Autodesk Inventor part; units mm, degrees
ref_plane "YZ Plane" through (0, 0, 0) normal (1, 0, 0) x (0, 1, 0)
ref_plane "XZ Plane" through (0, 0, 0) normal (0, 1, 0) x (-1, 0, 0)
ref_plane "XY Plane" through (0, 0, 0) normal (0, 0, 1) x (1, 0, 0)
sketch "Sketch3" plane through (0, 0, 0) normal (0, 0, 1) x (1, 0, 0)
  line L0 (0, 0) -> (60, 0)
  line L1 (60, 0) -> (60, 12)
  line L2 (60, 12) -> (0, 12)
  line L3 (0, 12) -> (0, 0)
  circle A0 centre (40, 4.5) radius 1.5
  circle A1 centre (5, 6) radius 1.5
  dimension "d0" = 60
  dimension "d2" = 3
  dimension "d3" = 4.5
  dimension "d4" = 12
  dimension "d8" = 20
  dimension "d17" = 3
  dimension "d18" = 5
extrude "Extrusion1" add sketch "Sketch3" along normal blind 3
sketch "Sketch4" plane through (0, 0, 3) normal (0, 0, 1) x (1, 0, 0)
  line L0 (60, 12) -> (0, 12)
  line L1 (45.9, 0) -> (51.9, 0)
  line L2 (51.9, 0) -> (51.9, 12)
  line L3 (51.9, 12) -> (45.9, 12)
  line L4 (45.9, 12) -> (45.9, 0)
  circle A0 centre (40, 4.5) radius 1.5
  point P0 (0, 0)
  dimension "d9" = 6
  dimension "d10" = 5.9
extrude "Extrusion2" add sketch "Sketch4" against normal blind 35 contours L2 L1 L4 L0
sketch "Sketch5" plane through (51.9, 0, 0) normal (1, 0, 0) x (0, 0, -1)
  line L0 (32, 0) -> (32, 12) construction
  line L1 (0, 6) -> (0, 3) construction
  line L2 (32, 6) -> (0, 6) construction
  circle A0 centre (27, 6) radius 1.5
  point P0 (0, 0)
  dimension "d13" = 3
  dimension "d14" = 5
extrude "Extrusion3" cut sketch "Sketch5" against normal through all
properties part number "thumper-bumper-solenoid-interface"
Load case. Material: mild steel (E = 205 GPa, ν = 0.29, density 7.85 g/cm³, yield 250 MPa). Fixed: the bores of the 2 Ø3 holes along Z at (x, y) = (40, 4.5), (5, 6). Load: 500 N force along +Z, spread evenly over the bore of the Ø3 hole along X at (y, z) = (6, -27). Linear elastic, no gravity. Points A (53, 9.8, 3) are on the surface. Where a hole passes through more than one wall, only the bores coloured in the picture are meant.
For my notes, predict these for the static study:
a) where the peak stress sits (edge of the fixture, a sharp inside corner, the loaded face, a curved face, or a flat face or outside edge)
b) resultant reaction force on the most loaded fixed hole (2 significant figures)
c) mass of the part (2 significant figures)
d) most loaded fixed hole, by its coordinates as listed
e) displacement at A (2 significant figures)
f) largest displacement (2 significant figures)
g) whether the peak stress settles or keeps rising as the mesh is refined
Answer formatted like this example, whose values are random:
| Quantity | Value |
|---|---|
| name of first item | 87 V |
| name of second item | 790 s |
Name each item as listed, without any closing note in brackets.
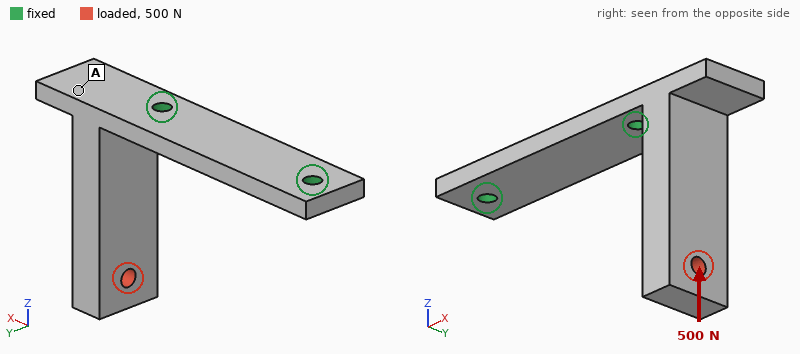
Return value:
| Quantity | Value |
|---|---|
| where the peak stress sits | edge of the fixture |
| resultant reaction force on the most loaded fixed hole | 510 N |
| mass of the part | 34 g |
| most loaded fixed hole, by its coordinates as listed | (40, 4.5) |
| displacement at A | 0.037 mm |
| largest displacement | 0.12 mm |
| whether the peak stress settles or keeps rising as the mesh is refined | keeps rising |
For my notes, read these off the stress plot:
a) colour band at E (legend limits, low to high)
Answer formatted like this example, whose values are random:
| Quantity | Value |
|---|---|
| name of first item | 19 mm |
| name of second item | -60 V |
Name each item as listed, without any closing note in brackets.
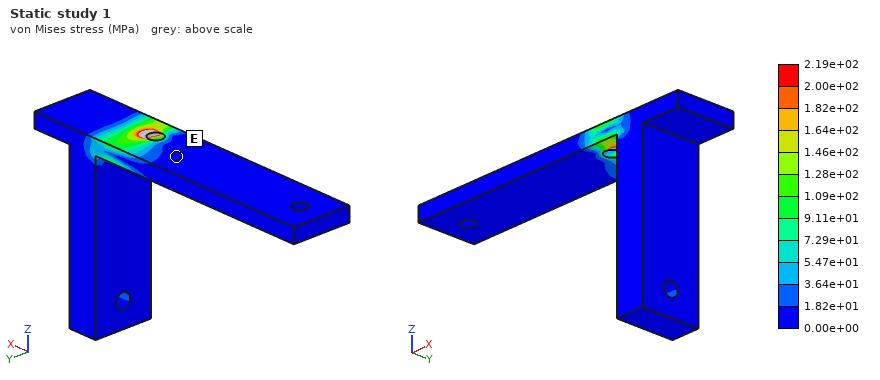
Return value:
| Quantity | Value |
|---|---|
| colour band at E | 0.00e+00 to 1.82e+01 MPa |
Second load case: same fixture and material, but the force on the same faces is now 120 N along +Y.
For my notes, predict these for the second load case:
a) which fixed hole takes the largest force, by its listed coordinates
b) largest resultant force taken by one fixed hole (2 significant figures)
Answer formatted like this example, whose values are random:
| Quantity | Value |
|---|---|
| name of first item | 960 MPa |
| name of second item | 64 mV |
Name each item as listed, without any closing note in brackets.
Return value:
| Quantity | Value |
|---|---|
| which fixed hole takes the largest force, by its listed coordinates | (40, 4.5) |
| largest resultant force taken by one fixed hole | 140 N |
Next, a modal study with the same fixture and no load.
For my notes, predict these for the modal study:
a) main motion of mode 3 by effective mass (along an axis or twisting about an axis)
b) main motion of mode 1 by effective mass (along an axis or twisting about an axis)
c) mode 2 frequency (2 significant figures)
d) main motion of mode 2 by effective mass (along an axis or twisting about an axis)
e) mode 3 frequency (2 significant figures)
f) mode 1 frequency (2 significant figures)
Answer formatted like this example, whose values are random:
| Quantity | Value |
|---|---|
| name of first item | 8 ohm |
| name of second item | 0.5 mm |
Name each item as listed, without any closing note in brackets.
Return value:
| Quantity | Value |
|---|---|
| main motion of mode 3 by effective mass | along Z |
| main motion of mode 1 by effective mass | along X |
| mode 2 frequency | 2200 Hz |
| main motion of mode 2 by effective mass | along Y |
| mode 3 frequency | 9300 Hz |
| mode 1 frequency | 1500 Hz |
